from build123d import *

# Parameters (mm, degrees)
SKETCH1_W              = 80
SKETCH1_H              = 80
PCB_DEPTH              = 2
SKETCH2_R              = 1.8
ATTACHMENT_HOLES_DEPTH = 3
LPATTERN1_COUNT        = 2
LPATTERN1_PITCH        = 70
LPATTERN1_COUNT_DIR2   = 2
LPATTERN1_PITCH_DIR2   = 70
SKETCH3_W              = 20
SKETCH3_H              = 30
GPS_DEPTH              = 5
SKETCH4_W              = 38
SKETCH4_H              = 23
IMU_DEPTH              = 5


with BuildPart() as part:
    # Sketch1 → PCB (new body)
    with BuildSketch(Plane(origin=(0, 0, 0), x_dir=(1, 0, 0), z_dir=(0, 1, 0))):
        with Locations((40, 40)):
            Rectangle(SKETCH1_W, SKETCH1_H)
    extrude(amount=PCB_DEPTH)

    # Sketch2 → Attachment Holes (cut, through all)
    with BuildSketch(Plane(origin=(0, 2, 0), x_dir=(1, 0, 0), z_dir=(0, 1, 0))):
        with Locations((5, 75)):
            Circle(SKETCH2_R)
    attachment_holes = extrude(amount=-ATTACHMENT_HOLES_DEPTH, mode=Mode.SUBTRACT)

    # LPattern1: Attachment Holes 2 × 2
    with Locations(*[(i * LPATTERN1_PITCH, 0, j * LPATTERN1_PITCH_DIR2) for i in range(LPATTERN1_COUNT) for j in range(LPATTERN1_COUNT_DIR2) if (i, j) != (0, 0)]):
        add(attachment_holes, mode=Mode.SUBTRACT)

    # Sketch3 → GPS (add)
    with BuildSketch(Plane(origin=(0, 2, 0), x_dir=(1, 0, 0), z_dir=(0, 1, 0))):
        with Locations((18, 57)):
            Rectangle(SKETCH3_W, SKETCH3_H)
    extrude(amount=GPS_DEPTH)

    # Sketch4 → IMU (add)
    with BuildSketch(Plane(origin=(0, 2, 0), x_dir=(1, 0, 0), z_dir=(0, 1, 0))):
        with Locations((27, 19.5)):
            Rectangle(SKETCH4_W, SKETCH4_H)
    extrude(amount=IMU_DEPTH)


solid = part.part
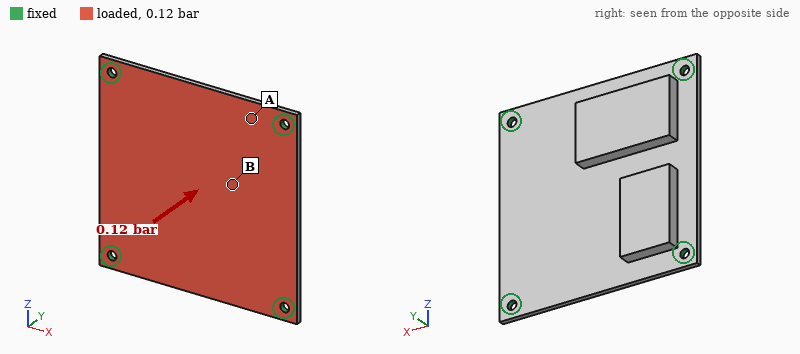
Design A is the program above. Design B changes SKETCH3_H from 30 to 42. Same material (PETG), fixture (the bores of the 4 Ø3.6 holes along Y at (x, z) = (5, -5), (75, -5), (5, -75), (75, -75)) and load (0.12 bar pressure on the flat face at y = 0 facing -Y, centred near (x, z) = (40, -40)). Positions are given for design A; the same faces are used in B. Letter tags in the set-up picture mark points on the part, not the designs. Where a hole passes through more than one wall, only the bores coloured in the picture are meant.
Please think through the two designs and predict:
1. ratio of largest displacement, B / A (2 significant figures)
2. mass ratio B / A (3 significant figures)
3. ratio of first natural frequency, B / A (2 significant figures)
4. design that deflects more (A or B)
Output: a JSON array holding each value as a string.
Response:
["0.90", "1.06", "1.0", "A"]
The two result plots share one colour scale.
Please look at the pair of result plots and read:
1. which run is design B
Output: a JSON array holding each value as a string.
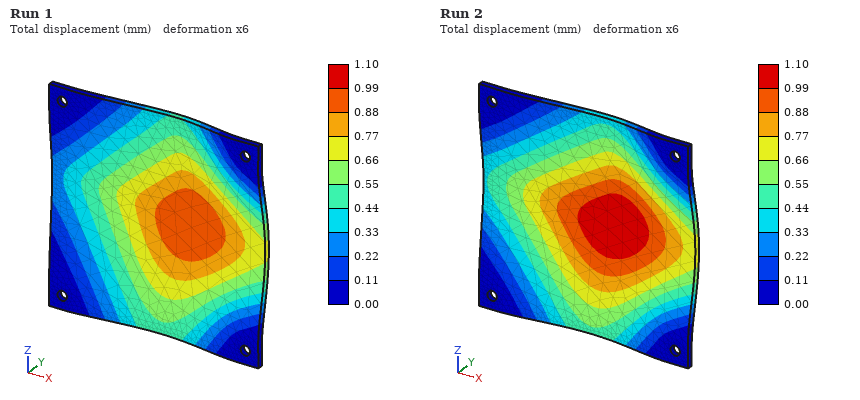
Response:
["Run 1"]
